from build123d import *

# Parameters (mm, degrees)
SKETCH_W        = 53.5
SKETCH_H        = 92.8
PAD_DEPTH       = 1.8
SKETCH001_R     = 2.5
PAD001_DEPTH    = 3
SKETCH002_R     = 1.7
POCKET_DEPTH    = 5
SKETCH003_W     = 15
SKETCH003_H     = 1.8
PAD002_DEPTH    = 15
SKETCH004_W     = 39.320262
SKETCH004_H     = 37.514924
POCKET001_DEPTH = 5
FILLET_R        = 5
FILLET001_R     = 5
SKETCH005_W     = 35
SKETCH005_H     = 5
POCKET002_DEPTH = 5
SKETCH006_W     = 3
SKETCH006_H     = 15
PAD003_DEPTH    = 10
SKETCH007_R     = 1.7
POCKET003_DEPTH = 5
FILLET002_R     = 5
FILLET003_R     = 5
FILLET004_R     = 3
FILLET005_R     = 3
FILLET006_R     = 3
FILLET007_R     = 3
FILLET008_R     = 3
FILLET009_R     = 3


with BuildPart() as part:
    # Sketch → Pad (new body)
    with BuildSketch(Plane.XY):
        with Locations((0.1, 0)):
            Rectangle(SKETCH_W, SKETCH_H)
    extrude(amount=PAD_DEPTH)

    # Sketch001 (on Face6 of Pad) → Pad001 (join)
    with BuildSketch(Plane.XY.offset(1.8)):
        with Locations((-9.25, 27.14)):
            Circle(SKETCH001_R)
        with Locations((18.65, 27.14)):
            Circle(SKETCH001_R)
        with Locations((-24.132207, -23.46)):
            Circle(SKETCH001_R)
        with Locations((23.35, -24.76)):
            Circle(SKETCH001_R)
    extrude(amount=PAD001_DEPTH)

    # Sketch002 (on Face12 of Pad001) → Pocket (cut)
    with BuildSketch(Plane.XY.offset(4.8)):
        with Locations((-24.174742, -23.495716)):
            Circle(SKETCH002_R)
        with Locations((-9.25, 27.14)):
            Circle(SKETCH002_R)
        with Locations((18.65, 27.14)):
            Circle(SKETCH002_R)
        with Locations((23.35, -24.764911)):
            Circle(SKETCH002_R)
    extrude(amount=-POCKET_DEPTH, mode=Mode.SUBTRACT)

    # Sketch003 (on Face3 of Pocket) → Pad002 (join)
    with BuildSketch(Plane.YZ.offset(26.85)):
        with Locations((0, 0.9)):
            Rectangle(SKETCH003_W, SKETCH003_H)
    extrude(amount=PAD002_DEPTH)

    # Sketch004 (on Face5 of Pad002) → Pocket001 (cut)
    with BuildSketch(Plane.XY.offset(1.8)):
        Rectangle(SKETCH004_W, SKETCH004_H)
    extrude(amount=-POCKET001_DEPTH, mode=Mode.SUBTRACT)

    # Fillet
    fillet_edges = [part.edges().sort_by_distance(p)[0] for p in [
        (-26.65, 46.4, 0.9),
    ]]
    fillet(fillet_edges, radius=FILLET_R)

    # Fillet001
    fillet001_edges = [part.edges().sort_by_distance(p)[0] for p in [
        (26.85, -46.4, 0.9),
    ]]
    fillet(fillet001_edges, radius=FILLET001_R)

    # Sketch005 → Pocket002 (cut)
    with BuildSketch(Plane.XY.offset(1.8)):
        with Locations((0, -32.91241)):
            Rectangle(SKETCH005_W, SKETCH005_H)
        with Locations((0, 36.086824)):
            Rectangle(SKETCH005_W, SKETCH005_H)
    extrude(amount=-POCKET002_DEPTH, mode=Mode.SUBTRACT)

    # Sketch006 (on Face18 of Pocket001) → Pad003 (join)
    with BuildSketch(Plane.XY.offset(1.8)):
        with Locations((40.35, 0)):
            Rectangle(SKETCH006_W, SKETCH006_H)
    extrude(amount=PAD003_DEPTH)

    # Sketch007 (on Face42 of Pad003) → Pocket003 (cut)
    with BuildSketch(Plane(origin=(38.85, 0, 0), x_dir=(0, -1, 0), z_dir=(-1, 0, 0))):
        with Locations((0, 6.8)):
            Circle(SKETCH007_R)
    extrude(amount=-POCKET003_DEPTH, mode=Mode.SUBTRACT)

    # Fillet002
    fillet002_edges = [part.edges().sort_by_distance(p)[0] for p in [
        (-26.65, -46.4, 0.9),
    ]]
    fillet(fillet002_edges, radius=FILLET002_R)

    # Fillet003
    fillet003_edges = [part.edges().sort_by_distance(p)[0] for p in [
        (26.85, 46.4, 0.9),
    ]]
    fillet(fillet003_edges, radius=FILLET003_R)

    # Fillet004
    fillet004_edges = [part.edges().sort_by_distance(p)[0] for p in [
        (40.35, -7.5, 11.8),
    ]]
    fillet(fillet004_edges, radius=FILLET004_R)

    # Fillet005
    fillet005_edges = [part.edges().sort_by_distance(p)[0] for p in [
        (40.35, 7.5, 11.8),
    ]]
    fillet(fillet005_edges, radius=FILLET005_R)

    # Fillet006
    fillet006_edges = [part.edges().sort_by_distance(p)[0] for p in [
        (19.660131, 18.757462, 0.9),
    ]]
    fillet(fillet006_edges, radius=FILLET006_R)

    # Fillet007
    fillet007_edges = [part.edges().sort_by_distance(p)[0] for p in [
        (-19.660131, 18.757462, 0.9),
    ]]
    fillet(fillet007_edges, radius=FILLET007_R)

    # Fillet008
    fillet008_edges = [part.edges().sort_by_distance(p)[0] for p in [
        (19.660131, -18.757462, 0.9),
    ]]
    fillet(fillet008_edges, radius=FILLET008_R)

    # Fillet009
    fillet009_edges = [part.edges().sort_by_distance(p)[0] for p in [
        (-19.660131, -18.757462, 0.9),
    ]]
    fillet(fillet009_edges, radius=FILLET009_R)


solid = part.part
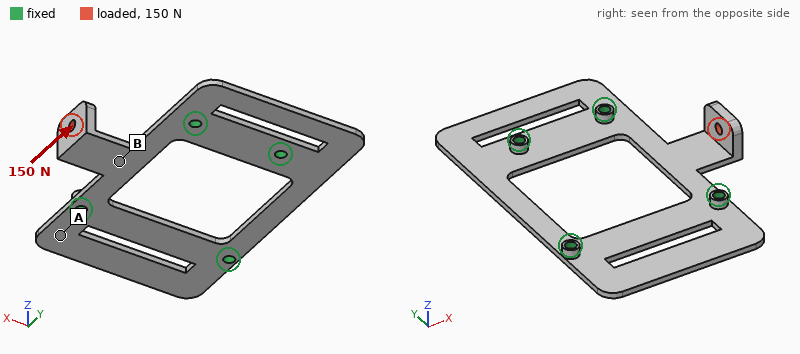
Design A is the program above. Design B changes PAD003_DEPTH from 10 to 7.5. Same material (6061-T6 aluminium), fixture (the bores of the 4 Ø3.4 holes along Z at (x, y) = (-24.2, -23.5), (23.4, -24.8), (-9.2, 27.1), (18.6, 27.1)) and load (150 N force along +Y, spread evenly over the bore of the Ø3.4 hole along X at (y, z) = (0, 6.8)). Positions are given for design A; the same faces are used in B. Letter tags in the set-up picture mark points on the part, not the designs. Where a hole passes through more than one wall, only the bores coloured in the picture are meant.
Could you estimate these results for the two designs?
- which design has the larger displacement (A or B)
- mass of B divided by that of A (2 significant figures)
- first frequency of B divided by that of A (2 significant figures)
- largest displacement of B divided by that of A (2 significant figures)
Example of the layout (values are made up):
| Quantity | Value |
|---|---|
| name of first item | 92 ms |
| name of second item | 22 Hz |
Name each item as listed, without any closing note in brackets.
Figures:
| Quantity | Value |
|---|---|
| which design has the larger displacement | A |
| mass of B divided by that of A | 0.98 |
| first frequency of B divided by that of A | 1.1 |
| largest displacement of B divided by that of A | 0.87 |
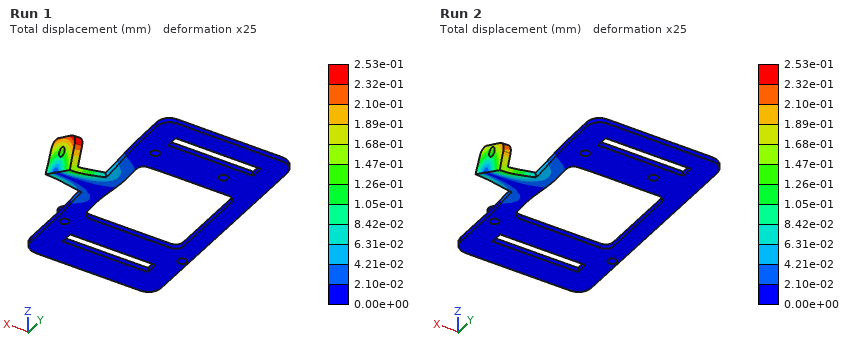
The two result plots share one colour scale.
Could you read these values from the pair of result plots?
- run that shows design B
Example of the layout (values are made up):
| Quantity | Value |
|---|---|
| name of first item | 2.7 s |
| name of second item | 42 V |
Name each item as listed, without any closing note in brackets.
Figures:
| Quantity | Value |
|---|---|
| run that shows design B | Run 2 |
